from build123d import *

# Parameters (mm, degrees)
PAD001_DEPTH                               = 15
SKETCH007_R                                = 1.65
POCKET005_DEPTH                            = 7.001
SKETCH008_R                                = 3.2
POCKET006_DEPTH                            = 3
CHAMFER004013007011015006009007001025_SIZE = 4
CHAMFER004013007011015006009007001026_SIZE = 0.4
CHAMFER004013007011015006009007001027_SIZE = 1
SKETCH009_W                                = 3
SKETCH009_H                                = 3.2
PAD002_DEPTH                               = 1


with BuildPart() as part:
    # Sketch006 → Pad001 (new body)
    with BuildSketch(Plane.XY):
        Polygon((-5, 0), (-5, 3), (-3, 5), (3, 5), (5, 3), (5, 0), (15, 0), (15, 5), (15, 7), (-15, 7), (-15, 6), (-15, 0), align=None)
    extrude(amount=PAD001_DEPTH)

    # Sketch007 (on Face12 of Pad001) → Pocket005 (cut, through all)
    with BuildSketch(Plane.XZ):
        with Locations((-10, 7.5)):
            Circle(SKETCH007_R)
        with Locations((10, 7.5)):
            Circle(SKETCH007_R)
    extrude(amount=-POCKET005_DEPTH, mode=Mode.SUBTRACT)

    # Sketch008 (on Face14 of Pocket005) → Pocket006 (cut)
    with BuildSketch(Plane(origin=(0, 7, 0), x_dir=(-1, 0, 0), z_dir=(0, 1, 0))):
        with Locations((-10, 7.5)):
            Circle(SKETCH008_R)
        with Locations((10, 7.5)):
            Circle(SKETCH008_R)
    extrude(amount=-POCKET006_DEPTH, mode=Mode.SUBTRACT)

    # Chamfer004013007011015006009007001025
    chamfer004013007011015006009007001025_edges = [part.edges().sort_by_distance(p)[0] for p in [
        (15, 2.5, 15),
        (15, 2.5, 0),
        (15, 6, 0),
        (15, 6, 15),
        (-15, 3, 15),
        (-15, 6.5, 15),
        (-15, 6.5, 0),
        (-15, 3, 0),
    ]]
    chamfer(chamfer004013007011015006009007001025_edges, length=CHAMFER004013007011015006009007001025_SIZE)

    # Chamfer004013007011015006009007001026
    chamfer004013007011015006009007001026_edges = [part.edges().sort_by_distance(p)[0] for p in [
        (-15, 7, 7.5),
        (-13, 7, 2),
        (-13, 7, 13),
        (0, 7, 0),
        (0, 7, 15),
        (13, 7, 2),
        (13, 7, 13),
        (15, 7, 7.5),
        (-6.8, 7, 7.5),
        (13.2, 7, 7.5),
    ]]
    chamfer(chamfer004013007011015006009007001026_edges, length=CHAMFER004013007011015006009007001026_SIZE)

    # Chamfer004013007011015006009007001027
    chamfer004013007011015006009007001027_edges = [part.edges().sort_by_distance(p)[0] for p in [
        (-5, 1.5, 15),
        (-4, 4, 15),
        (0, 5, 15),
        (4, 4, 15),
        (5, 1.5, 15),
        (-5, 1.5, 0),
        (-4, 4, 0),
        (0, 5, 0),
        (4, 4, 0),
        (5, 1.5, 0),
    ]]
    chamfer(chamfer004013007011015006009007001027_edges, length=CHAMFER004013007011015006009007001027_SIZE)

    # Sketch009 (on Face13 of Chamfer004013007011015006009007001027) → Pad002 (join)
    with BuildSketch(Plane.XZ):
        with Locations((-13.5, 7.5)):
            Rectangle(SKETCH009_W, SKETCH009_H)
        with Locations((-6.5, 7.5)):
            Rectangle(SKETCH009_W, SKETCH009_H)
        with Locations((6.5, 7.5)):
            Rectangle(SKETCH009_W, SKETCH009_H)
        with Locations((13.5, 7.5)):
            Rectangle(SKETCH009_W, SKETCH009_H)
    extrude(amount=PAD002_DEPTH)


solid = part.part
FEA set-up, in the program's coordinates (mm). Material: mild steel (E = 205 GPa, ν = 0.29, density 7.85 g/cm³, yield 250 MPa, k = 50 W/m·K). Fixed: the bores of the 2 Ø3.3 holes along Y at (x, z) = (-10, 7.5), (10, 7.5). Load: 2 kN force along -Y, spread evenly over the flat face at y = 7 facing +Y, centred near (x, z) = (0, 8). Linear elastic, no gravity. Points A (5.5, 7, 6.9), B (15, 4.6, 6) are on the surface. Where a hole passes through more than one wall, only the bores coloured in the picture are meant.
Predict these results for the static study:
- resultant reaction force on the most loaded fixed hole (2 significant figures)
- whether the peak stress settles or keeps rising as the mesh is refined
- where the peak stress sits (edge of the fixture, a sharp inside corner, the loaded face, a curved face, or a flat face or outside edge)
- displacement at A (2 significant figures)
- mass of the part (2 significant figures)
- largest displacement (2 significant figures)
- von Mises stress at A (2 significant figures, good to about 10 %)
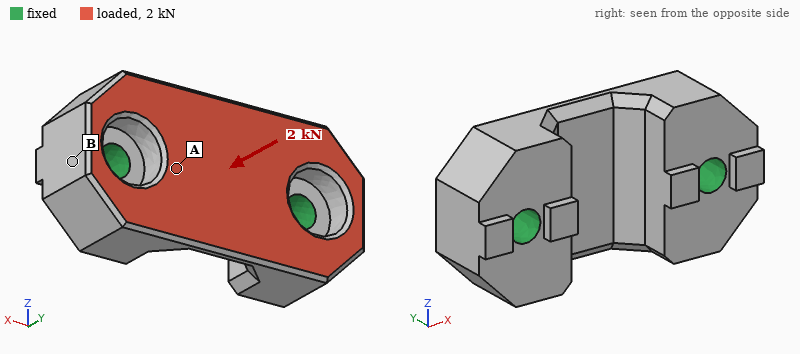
1.1 kN
keeps rising
edge of the fixture
1.6 µm
16 g
3.7 µm
25 MPa
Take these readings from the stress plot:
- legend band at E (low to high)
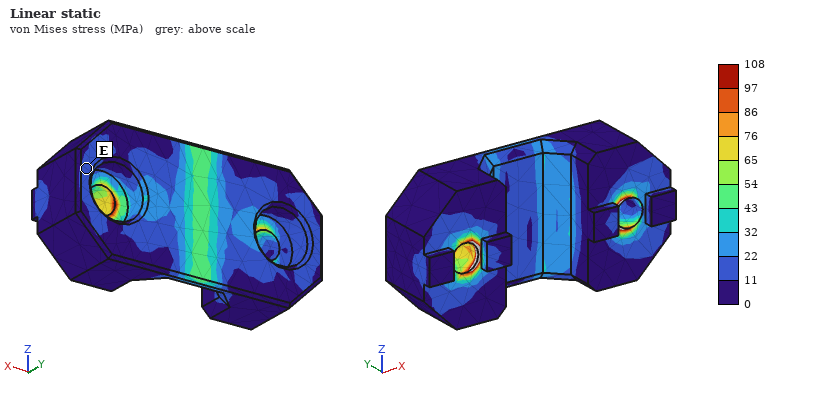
11 to 22 MPa
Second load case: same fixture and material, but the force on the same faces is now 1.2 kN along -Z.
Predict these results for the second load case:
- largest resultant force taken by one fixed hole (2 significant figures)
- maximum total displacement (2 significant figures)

600 N
5.2 µm
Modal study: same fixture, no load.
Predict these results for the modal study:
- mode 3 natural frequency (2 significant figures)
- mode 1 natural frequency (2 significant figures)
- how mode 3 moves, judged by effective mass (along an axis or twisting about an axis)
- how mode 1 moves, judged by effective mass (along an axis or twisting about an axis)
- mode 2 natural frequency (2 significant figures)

52 kHz
33 kHz
along Y
along Z
43 kHz
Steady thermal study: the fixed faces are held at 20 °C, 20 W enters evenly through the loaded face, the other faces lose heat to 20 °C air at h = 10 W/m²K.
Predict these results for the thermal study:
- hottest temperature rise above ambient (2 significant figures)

25 K
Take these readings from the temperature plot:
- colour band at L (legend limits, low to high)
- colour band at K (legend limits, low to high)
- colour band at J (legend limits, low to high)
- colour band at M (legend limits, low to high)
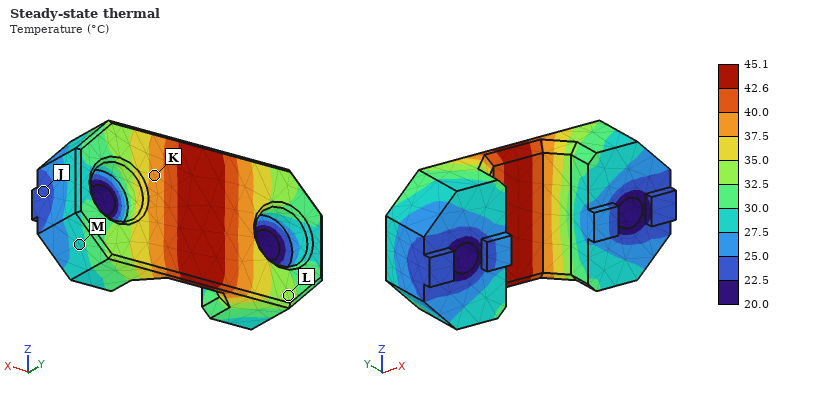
32.5 to 35.0 °C
37.5 to 40.0 °C
22.5 to 25.0 °C
27.5 to 30.0 °C
